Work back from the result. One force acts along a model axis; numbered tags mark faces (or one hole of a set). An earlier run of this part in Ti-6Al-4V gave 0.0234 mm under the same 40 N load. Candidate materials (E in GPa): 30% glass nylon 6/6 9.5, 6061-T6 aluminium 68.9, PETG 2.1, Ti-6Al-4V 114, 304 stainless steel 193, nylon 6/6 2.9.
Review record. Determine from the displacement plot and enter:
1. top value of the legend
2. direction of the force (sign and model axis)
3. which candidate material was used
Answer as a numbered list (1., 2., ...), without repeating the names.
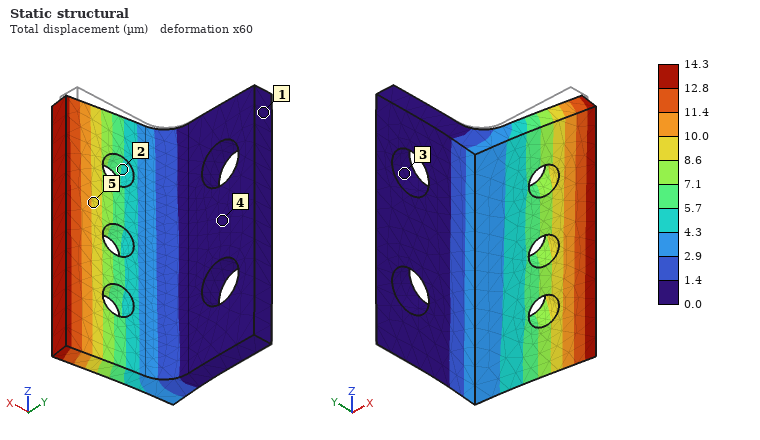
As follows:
1. 14.3 µm
2. -Y
3. 304 stainless steel
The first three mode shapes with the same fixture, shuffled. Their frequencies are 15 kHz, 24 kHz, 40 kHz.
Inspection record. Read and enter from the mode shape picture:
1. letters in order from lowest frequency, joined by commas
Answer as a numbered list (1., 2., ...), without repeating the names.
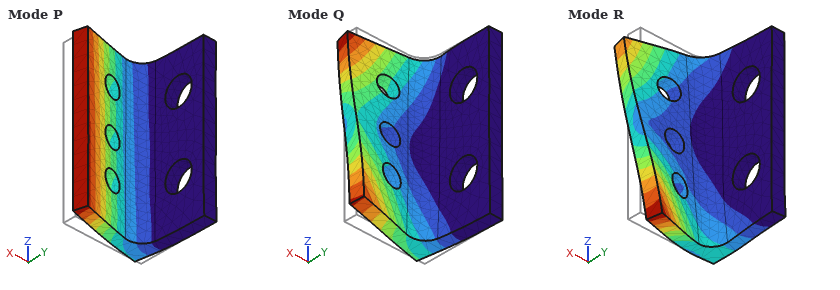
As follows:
1. P, Q, R
